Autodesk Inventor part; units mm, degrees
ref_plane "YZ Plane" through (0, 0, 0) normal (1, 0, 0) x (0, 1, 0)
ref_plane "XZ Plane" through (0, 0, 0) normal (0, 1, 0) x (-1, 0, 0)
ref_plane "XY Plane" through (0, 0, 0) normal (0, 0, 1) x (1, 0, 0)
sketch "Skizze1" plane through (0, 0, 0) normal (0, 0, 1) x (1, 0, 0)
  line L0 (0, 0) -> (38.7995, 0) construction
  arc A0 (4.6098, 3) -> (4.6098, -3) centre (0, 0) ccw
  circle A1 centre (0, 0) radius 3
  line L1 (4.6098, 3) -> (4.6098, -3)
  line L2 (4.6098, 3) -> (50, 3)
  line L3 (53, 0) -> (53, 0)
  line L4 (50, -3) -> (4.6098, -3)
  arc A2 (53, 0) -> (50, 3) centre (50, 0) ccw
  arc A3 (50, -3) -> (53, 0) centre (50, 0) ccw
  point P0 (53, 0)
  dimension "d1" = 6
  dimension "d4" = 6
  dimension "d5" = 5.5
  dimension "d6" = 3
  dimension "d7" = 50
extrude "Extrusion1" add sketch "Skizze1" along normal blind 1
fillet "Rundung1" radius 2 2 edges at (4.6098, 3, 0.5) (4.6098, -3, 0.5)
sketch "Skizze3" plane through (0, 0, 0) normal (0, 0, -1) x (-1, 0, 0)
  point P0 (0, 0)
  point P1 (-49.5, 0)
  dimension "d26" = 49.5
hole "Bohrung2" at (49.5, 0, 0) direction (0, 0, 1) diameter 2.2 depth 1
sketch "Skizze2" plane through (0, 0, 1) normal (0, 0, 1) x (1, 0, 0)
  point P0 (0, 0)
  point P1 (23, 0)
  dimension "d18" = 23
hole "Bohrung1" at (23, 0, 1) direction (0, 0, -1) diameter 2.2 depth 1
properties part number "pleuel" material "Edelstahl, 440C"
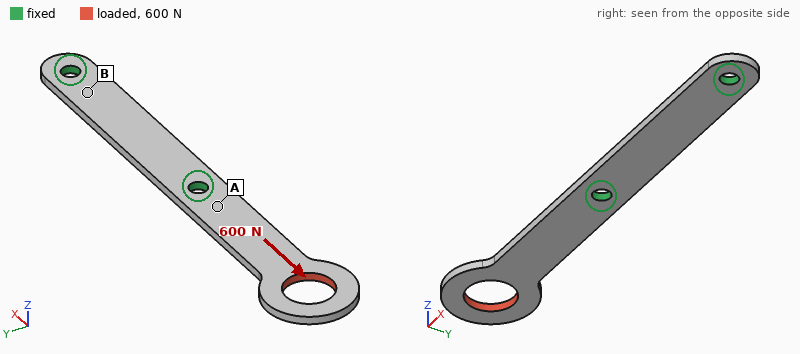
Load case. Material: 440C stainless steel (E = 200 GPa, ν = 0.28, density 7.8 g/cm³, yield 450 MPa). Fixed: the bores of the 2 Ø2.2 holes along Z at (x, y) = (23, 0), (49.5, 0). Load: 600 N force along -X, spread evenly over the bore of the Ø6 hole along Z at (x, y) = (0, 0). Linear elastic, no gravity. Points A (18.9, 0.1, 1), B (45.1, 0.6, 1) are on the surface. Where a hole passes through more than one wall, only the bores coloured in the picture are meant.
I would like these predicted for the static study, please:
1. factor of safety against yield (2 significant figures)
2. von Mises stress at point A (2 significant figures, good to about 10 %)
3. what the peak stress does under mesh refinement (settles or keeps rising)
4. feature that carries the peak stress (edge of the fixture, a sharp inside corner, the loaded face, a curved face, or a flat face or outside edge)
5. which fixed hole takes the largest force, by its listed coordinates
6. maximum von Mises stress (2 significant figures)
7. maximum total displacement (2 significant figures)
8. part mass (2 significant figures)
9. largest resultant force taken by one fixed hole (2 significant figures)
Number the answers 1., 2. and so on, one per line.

1. 1.4
2. 110 MPa
3. settles
4. a curved face
5. (23, 0)
6. 320 MPa
7. 19 µm
8. 2.7 g
9. 590 N
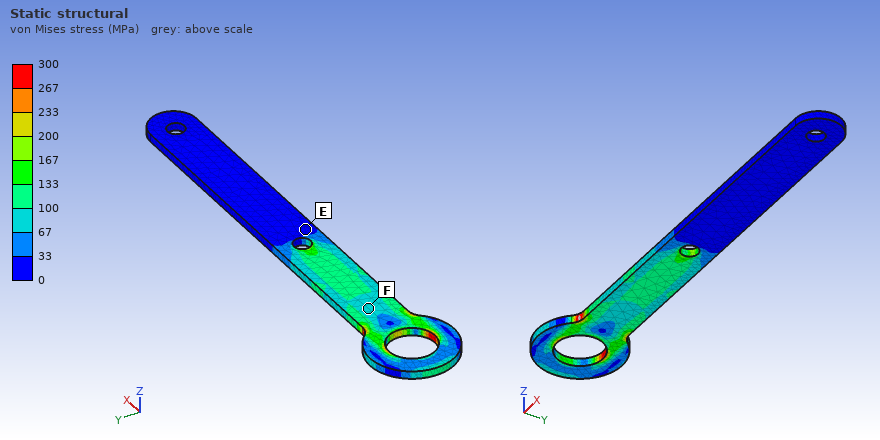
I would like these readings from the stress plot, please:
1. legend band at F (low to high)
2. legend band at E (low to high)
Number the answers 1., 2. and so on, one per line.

1. 67 to 100 MPa
2. 0 to 33 MPa
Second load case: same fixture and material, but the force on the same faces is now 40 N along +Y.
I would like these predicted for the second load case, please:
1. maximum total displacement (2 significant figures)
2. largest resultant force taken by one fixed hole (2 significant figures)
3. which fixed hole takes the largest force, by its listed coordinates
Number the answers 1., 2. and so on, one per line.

1. 77 µm
2. 50 N
3. (23, 0)
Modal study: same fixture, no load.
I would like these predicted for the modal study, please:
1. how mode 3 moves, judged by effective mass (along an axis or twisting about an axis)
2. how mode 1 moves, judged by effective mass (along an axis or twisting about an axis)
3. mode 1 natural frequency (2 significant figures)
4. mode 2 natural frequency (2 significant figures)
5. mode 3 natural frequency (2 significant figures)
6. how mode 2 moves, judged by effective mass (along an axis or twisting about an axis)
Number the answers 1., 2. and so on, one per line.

1. twisting about X
2. along Z
3. 1100 Hz
4. 5200 Hz
5. 5500 Hz
6. along Y
